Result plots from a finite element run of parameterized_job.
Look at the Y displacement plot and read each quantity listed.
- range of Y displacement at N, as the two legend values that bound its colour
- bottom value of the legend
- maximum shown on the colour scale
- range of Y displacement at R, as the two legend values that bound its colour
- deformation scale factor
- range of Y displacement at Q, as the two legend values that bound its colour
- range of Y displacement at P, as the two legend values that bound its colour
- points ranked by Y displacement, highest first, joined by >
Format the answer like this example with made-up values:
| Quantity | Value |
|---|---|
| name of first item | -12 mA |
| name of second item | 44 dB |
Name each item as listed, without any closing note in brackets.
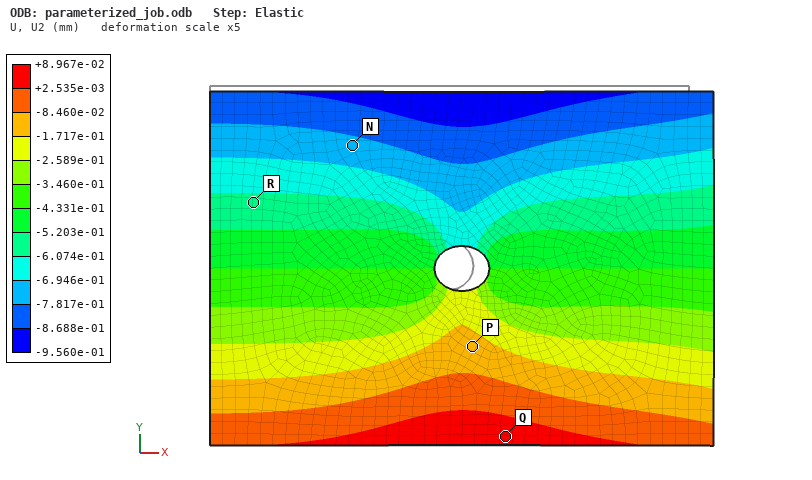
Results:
| Quantity | Value |
|---|---|
| range of Y displacement at N, as the two legend values that bound its colour | -7.817e-01 to -6.946e-01 mm |
| bottom value of the legend | -9.560e-01 mm |
| maximum shown on the colour scale | +8.967e-02 mm |
| range of Y displacement at R, as the two legend values that bound its colour | -6.074e-01 to -5.203e-01 mm |
| deformation scale factor | 5 |
| range of Y displacement at Q, as the two legend values that bound its colour | +2.535e-03 to +8.967e-02 mm |
| range of Y displacement at P, as the two legend values that bound its colour | -1.717e-01 to -8.460e-02 mm |
| points ranked by Y displacement, highest first, joined by > | Q > P > R > N |
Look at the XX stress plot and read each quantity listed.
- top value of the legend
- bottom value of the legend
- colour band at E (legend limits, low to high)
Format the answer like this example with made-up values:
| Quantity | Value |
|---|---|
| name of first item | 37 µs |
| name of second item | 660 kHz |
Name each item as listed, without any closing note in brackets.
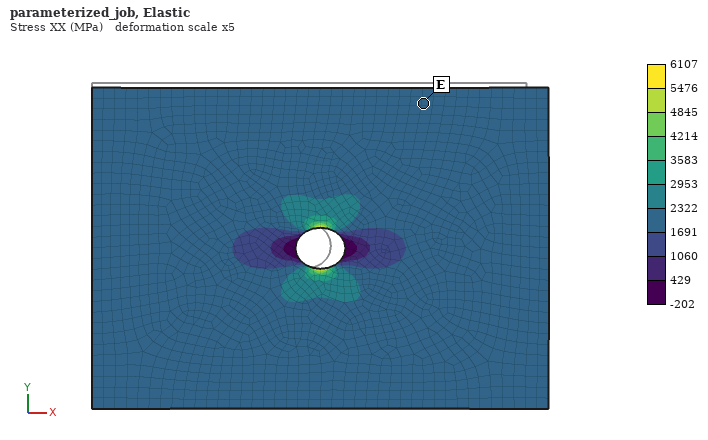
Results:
| Quantity | Value |
|---|---|
| top value of the legend | 6107 MPa |
| bottom value of the legend | -202 MPa |
| colour band at E | 1691 to 2322 MPa |
